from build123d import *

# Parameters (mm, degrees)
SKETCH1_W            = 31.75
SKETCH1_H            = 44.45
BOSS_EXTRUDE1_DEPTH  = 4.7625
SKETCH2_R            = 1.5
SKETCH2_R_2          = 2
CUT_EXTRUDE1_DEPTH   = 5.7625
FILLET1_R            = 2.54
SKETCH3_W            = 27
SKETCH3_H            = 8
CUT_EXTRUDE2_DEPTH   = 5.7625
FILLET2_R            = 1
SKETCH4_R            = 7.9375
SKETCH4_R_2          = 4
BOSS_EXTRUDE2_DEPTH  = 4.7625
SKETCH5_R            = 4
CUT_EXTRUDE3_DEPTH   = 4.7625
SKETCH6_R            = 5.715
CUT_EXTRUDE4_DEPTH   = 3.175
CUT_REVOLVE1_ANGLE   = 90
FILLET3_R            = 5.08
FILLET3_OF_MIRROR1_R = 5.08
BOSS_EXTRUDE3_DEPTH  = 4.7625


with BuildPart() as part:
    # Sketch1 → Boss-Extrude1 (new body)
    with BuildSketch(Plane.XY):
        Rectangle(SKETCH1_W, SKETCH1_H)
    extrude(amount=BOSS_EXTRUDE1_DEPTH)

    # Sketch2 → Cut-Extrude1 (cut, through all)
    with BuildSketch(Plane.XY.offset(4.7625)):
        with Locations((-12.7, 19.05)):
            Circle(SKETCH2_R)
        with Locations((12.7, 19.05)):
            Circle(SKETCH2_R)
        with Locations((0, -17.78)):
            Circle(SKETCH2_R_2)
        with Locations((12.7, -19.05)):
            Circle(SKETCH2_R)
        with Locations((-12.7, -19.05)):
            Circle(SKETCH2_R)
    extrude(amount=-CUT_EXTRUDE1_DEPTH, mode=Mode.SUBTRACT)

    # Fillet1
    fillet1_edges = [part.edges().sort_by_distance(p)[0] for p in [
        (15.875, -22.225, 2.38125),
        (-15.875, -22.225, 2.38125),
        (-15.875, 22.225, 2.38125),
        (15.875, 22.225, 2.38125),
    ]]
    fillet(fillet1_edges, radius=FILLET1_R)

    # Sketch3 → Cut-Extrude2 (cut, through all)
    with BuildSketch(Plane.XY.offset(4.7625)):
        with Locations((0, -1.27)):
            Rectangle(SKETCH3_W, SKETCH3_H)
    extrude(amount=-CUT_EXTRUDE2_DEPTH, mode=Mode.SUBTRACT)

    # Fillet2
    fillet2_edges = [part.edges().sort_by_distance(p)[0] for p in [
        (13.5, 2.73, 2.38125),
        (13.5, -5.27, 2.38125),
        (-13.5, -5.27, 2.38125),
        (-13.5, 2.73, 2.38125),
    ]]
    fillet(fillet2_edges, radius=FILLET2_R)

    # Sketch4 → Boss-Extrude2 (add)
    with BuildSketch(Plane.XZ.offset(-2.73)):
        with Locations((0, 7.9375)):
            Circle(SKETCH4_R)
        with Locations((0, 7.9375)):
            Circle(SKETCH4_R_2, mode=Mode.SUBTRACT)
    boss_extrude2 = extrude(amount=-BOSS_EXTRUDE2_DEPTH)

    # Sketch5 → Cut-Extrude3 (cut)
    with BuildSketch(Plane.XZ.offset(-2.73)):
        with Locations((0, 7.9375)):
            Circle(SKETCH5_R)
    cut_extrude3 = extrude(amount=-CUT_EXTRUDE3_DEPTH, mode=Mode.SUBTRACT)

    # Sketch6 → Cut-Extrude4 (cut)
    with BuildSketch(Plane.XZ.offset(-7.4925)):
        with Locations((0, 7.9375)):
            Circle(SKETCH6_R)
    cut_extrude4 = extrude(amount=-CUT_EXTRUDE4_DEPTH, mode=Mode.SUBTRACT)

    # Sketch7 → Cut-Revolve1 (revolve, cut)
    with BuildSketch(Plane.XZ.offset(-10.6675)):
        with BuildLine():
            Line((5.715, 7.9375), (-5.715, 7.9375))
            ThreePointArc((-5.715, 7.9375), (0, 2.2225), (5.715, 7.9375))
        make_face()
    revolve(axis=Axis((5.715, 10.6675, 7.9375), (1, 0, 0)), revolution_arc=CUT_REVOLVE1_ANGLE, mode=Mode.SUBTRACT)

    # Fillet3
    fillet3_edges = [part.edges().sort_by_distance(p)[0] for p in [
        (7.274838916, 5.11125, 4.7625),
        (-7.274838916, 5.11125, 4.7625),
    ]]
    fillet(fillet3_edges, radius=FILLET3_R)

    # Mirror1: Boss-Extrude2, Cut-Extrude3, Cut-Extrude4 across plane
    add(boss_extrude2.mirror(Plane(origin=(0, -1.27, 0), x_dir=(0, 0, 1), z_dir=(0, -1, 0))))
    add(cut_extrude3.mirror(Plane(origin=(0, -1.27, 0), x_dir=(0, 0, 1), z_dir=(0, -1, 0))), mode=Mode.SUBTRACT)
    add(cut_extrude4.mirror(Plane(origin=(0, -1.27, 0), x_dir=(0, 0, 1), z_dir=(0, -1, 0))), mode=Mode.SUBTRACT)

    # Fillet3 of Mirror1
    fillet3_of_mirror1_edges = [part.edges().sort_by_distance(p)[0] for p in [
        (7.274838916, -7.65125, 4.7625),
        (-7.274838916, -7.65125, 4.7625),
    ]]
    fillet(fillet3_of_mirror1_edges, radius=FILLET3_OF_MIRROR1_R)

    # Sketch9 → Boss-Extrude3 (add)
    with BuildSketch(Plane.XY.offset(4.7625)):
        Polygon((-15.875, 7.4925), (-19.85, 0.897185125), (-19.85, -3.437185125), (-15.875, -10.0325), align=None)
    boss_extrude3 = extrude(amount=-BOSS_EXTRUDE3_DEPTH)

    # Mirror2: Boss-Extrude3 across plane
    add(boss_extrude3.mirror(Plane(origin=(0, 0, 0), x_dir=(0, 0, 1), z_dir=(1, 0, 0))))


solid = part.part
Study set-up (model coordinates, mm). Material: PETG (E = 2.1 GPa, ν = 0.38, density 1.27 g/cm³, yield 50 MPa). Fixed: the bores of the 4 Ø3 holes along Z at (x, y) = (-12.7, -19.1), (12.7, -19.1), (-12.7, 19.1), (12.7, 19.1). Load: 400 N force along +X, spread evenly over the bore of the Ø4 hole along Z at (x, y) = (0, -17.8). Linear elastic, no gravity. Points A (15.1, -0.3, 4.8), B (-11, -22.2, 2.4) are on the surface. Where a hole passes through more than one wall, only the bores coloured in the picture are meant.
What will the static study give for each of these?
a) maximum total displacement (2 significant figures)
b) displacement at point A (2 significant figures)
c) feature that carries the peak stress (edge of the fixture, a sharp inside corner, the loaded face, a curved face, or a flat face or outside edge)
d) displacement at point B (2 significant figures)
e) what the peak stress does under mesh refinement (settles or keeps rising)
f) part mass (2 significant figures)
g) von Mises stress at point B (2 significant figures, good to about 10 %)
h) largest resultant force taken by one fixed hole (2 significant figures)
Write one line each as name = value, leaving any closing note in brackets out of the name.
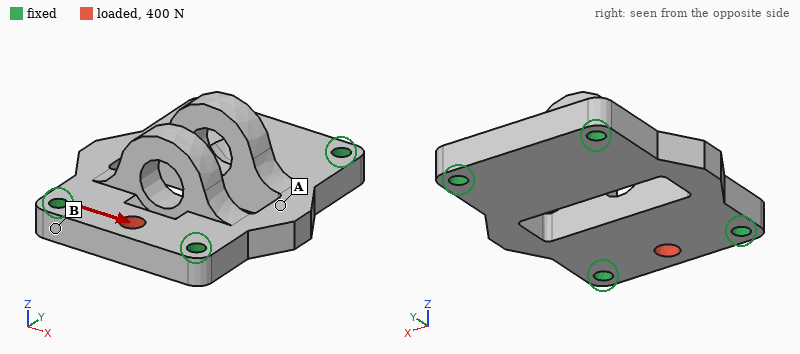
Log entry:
maximum total displacement = 31 µm
displacement at point A = 8.7 µm
feature that carries the peak stress = edge of the fixture
displacement at point B = 5.9 µm
what the peak stress does under mesh refinement = keeps rising
part mass = 8.6 g
von Mises stress at point B = 2.8 MPa
largest resultant force taken by one fixed hole = 200 N
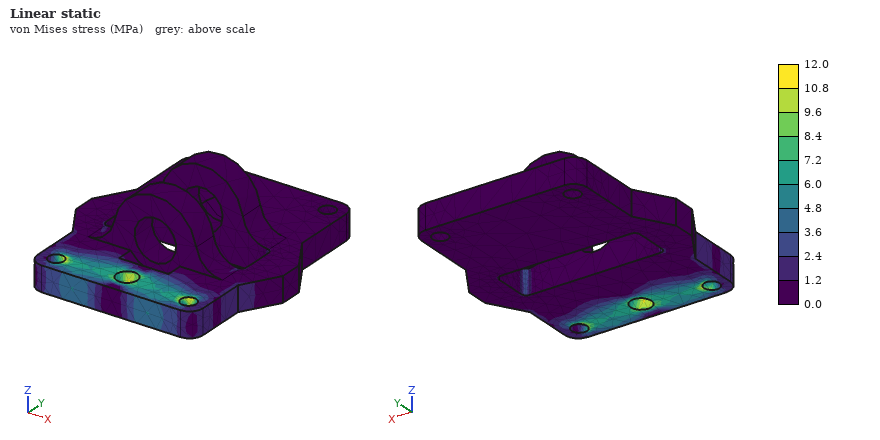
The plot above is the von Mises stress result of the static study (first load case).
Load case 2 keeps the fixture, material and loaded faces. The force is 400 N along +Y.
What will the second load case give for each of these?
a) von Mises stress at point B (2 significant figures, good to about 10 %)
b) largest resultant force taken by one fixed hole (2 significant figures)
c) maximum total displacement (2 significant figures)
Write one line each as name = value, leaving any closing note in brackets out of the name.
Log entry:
von Mises stress at point B = 6.7 MPa
largest resultant force taken by one fixed hole = 210 N
maximum total displacement = 93 µm
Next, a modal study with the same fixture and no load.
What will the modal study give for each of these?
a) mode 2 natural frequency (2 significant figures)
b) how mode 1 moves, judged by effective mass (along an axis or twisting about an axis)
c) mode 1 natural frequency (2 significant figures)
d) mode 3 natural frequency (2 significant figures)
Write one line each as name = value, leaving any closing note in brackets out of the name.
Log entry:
mode 2 natural frequency = 3800 Hz
how mode 1 moves, judged by effective mass = along Z
mode 1 natural frequency = 2500 Hz
mode 3 natural frequency = 3800 Hz
